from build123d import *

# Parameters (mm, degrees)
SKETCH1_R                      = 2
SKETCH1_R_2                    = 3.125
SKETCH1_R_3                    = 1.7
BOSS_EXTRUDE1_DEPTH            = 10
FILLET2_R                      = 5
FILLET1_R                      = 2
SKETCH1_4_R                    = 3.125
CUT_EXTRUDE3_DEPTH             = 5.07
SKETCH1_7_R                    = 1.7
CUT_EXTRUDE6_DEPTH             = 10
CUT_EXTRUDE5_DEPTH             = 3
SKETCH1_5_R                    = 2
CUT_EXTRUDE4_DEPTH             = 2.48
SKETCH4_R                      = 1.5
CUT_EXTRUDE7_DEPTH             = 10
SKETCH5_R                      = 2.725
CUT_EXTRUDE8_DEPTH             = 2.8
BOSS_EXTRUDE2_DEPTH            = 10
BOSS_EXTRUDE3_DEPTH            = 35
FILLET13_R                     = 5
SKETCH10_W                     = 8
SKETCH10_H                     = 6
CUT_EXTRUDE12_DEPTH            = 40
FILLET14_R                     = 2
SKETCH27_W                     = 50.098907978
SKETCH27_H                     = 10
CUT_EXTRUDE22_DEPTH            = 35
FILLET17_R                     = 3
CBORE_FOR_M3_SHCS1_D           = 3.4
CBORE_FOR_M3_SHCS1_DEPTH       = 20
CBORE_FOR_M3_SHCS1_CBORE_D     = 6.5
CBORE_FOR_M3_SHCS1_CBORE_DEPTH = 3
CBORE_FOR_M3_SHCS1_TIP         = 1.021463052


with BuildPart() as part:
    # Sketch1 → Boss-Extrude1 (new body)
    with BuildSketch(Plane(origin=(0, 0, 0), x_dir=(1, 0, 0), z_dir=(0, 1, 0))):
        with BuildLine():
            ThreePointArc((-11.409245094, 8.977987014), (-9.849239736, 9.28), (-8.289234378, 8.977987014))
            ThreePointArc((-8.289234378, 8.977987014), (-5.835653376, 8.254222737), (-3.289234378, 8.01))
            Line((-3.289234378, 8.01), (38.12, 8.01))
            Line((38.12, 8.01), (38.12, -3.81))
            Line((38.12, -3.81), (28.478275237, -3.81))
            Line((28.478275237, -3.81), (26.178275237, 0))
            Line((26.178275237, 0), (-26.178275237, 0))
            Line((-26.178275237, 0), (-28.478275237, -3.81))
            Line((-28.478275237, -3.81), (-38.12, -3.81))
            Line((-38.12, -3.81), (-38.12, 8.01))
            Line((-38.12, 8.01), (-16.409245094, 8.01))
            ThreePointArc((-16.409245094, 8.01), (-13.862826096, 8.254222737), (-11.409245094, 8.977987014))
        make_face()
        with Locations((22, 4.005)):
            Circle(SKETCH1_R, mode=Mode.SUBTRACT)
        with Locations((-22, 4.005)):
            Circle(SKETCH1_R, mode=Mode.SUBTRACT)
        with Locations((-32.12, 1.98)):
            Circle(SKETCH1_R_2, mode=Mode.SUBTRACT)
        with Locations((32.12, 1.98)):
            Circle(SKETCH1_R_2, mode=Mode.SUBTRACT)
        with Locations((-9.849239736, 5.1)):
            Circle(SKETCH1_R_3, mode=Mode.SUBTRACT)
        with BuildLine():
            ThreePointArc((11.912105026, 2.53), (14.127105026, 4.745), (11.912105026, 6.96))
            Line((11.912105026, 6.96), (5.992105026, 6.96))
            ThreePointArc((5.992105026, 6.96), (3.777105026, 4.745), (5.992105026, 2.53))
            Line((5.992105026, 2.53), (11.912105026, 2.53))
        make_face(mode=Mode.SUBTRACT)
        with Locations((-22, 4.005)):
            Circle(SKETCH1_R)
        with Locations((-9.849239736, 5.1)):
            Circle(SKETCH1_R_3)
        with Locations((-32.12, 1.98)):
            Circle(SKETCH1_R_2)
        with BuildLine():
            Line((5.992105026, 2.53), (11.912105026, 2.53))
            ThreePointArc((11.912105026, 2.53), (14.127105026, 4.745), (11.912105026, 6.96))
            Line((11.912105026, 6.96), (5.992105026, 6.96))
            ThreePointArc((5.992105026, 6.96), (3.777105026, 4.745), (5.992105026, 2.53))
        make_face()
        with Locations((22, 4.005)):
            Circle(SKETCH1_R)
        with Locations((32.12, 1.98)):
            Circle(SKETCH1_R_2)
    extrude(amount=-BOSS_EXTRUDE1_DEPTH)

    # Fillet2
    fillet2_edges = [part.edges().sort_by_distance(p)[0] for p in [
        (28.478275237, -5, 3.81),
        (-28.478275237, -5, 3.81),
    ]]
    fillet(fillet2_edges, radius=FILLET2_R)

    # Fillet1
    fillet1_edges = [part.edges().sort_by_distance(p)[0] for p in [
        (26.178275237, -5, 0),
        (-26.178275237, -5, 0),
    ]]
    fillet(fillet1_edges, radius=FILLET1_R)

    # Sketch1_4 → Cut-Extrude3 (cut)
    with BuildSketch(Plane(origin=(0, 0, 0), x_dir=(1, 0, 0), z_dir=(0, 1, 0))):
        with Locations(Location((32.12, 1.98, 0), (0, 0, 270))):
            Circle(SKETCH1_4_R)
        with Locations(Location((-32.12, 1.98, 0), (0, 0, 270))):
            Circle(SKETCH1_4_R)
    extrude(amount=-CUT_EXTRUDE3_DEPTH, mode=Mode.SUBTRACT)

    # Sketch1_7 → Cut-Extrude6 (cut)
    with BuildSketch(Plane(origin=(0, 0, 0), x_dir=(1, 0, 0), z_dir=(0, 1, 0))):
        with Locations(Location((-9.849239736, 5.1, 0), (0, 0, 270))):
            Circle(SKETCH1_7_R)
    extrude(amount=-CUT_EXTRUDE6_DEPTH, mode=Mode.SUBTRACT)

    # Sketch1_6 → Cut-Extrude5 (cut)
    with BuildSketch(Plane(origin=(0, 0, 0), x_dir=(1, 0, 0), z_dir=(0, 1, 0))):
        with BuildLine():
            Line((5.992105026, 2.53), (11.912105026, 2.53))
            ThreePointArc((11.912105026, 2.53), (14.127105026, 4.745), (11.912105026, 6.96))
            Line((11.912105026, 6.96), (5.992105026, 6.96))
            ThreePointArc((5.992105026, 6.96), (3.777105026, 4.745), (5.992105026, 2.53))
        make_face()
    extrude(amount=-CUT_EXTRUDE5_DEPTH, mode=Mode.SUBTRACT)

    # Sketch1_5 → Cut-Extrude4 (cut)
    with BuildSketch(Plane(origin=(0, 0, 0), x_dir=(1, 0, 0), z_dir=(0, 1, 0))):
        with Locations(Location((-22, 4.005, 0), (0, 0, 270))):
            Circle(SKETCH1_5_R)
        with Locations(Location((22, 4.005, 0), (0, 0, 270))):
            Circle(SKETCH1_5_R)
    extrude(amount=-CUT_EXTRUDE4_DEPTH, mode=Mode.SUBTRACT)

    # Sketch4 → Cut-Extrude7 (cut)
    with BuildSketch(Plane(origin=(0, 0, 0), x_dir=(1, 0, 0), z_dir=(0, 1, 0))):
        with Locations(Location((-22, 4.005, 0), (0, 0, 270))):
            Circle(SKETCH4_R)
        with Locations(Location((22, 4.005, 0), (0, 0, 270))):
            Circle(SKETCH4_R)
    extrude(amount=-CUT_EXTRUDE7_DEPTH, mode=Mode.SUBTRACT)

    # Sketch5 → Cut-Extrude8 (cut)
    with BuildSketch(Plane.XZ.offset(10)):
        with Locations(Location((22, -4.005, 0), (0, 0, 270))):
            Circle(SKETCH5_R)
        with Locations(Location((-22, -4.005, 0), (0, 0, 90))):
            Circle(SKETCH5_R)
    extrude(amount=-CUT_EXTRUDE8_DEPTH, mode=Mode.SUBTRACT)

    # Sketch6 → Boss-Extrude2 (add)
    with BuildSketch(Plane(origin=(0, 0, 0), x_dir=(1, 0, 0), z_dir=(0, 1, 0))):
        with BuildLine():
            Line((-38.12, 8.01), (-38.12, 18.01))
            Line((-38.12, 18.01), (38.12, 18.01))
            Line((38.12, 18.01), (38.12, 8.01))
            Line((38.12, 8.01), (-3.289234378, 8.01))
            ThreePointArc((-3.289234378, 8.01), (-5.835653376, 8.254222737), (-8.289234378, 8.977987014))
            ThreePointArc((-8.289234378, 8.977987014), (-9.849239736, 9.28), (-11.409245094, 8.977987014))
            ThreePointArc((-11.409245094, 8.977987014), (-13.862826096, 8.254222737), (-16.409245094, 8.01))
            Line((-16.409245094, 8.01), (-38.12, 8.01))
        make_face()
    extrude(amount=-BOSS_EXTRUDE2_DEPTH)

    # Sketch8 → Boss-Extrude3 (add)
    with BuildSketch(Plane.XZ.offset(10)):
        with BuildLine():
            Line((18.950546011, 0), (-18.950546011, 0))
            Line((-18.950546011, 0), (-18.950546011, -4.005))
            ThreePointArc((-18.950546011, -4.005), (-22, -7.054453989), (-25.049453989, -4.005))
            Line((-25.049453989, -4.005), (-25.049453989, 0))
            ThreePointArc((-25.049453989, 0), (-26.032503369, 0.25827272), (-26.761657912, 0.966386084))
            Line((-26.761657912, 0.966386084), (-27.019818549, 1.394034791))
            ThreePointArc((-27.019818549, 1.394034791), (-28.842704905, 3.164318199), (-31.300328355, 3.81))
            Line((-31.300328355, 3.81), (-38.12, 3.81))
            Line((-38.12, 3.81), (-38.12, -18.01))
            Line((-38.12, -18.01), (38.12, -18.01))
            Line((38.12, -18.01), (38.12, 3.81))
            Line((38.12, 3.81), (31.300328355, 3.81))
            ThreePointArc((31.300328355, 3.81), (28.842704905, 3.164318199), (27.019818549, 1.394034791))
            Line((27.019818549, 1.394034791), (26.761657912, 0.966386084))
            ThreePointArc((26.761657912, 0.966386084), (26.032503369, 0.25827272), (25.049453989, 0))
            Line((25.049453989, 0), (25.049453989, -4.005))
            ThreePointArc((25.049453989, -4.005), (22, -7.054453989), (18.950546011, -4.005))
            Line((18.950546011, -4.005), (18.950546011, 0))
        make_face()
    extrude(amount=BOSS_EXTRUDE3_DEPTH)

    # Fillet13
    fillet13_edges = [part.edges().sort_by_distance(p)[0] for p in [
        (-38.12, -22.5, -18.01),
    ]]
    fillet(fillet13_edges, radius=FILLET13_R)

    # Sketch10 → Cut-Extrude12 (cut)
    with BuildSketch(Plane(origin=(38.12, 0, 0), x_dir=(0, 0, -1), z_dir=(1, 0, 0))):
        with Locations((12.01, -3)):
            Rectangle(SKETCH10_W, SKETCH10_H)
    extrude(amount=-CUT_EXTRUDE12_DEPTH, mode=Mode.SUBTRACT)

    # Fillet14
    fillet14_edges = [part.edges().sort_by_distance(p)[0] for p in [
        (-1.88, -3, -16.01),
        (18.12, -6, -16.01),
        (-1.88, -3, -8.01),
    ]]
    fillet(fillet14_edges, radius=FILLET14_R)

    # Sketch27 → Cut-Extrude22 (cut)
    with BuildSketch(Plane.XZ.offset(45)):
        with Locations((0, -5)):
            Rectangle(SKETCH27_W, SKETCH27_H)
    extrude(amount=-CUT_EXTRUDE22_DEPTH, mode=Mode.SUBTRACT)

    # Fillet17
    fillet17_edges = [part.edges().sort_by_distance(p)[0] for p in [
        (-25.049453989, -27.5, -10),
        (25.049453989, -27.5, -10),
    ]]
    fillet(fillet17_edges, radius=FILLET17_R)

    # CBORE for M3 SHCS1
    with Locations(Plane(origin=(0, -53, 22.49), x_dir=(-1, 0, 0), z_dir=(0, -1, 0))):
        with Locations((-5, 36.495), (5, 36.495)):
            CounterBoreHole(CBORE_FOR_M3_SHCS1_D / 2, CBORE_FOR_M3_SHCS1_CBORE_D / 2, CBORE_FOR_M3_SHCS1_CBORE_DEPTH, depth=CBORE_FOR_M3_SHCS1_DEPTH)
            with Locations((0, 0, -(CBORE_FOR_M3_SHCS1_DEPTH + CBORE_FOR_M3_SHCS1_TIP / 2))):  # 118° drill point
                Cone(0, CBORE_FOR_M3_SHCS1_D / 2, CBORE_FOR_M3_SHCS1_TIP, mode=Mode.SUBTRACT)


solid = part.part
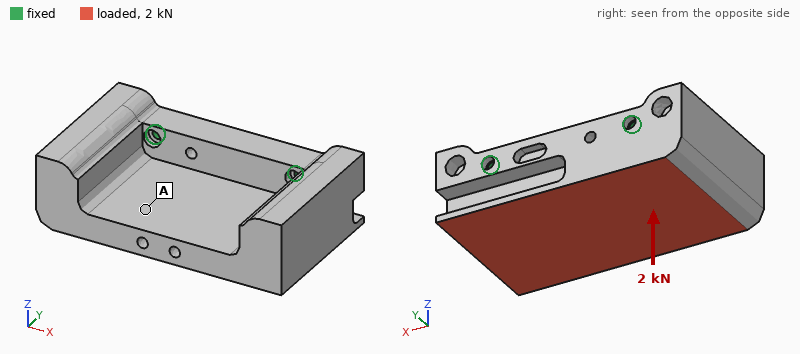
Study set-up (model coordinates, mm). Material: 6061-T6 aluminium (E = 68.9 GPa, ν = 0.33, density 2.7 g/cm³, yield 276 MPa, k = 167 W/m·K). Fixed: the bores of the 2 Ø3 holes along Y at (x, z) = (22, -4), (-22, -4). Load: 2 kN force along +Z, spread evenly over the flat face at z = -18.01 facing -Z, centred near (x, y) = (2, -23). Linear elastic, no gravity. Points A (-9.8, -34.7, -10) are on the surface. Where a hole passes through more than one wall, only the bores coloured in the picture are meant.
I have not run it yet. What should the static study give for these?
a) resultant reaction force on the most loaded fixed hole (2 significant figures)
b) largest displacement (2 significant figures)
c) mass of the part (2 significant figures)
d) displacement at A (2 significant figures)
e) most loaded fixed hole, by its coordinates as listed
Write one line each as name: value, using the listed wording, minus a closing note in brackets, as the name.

resultant reaction force on the most loaded fixed hole: 1.1 kN
largest displacement: 0.25 mm
mass of the part: 120 g
displacement at A: 0.17 mm
most loaded fixed hole, by its coordinates as listed: (22, -4)
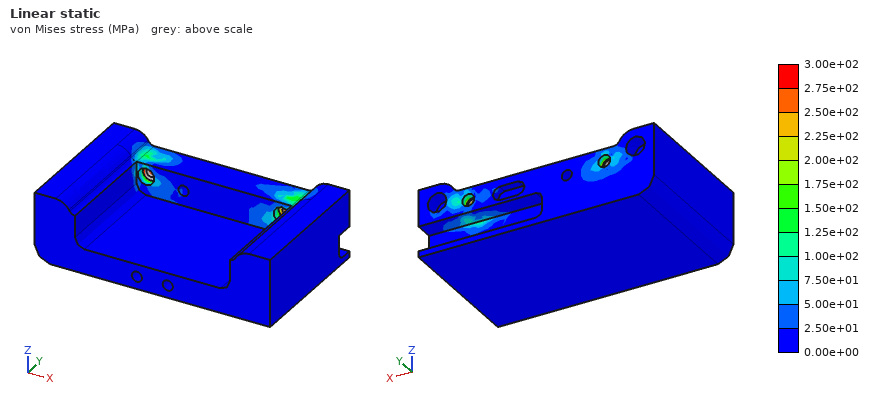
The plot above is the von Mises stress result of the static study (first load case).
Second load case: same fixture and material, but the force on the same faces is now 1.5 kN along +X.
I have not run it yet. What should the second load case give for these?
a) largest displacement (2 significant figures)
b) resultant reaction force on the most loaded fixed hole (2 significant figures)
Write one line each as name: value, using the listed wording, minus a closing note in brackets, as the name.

largest displacement: 13 µm
resultant reaction force on the most loaded fixed hole: 1.1 kN
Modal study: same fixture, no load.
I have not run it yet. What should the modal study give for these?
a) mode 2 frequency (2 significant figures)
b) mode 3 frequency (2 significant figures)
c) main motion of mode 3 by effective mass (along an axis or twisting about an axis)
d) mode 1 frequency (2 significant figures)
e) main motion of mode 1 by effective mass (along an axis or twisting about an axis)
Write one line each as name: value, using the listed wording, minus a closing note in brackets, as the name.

mode 2 frequency: 3200 Hz
mode 3 frequency: 6600 Hz
main motion of mode 3 by effective mass: along X
mode 1 frequency: 1600 Hz
main motion of mode 1 by effective mass: along Z
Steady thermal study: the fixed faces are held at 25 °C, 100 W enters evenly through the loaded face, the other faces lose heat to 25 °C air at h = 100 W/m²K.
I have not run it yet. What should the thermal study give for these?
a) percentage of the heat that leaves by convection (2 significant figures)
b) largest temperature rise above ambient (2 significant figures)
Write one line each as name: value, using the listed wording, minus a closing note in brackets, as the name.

percentage of the heat that leaves by convection: 19 %
largest temperature rise above ambient: 28 K
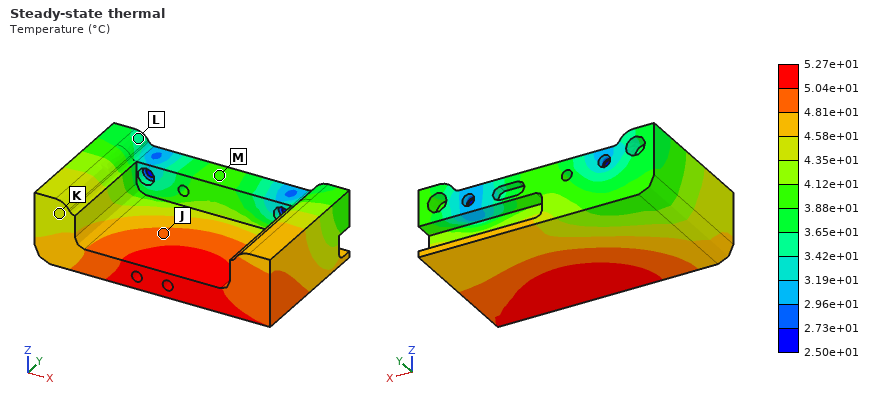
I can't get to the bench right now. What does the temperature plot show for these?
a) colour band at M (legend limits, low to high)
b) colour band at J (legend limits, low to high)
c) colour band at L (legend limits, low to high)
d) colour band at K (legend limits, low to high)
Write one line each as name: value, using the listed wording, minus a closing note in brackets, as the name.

colour band at M: 3.88e+01 to 4.12e+01 °C
colour band at J: 4.81e+01 to 5.04e+01 °C
colour band at L: 3.42e+01 to 3.65e+01 °C
colour band at K: 4.35e+01 to 4.58e+01 °C
